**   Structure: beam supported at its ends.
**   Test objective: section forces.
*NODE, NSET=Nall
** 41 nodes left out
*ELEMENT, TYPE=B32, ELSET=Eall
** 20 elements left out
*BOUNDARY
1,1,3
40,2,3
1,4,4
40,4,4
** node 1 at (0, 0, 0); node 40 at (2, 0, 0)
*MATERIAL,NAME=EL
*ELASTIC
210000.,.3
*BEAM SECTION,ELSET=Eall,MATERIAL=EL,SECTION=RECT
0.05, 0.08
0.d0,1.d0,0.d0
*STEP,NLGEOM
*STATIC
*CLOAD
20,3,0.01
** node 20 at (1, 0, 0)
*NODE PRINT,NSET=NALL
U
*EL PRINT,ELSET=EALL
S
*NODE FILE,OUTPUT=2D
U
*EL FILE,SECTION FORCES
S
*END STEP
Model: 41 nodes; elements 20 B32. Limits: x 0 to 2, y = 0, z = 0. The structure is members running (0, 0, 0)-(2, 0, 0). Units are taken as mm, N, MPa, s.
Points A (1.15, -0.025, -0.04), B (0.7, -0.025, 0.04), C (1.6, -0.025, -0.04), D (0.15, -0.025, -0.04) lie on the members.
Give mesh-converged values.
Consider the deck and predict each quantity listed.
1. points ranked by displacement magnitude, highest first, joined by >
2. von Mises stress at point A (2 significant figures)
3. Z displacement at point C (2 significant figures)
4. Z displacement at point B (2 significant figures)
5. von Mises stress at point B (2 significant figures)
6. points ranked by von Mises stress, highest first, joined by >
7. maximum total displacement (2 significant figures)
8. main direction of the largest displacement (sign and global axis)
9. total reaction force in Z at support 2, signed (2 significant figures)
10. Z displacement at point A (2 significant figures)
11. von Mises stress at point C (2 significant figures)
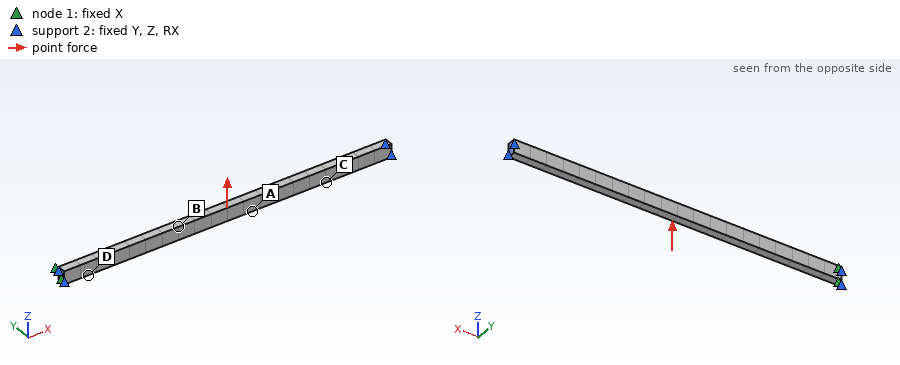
A > B > C > D
80 MPa
0.0021 mm
0.0033 mm
66 MPa
A > B > C > D
0.0037 mm
+Z
-0.010 N
0.0036 mm
38 MPa
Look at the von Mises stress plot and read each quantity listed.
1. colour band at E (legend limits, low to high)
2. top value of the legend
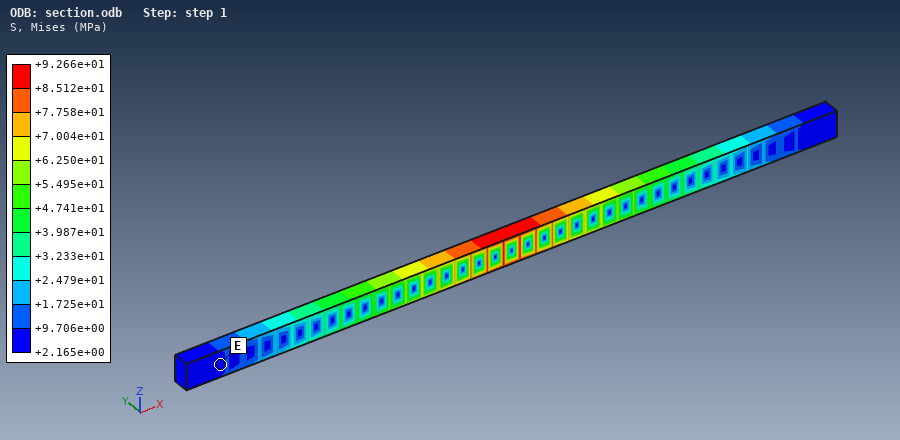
+2.165e+00 to +9.706e+00 MPa
+9.266e+01 MPa
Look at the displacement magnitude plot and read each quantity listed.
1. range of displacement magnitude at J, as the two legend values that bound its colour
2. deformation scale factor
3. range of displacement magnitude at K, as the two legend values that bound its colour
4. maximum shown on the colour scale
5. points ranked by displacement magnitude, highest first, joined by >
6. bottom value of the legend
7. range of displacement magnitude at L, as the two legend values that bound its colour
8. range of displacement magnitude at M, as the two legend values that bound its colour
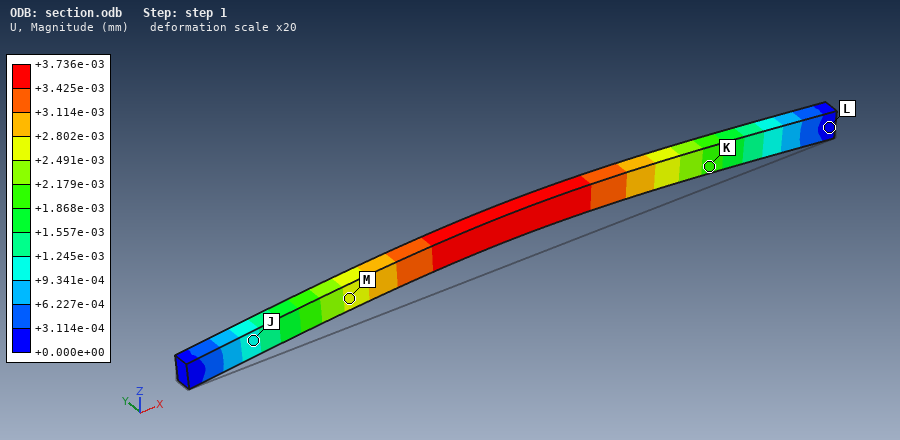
+9.341e-04 to +1.245e-03 mm
20
+1.868e-03 to +2.179e-03 mm
+3.736e-03 mm
M > K > J > L
+0.000e+00 mm
+0.000e+00 to +3.114e-04 mm
+2.491e-03 to +2.802e-03 mm
